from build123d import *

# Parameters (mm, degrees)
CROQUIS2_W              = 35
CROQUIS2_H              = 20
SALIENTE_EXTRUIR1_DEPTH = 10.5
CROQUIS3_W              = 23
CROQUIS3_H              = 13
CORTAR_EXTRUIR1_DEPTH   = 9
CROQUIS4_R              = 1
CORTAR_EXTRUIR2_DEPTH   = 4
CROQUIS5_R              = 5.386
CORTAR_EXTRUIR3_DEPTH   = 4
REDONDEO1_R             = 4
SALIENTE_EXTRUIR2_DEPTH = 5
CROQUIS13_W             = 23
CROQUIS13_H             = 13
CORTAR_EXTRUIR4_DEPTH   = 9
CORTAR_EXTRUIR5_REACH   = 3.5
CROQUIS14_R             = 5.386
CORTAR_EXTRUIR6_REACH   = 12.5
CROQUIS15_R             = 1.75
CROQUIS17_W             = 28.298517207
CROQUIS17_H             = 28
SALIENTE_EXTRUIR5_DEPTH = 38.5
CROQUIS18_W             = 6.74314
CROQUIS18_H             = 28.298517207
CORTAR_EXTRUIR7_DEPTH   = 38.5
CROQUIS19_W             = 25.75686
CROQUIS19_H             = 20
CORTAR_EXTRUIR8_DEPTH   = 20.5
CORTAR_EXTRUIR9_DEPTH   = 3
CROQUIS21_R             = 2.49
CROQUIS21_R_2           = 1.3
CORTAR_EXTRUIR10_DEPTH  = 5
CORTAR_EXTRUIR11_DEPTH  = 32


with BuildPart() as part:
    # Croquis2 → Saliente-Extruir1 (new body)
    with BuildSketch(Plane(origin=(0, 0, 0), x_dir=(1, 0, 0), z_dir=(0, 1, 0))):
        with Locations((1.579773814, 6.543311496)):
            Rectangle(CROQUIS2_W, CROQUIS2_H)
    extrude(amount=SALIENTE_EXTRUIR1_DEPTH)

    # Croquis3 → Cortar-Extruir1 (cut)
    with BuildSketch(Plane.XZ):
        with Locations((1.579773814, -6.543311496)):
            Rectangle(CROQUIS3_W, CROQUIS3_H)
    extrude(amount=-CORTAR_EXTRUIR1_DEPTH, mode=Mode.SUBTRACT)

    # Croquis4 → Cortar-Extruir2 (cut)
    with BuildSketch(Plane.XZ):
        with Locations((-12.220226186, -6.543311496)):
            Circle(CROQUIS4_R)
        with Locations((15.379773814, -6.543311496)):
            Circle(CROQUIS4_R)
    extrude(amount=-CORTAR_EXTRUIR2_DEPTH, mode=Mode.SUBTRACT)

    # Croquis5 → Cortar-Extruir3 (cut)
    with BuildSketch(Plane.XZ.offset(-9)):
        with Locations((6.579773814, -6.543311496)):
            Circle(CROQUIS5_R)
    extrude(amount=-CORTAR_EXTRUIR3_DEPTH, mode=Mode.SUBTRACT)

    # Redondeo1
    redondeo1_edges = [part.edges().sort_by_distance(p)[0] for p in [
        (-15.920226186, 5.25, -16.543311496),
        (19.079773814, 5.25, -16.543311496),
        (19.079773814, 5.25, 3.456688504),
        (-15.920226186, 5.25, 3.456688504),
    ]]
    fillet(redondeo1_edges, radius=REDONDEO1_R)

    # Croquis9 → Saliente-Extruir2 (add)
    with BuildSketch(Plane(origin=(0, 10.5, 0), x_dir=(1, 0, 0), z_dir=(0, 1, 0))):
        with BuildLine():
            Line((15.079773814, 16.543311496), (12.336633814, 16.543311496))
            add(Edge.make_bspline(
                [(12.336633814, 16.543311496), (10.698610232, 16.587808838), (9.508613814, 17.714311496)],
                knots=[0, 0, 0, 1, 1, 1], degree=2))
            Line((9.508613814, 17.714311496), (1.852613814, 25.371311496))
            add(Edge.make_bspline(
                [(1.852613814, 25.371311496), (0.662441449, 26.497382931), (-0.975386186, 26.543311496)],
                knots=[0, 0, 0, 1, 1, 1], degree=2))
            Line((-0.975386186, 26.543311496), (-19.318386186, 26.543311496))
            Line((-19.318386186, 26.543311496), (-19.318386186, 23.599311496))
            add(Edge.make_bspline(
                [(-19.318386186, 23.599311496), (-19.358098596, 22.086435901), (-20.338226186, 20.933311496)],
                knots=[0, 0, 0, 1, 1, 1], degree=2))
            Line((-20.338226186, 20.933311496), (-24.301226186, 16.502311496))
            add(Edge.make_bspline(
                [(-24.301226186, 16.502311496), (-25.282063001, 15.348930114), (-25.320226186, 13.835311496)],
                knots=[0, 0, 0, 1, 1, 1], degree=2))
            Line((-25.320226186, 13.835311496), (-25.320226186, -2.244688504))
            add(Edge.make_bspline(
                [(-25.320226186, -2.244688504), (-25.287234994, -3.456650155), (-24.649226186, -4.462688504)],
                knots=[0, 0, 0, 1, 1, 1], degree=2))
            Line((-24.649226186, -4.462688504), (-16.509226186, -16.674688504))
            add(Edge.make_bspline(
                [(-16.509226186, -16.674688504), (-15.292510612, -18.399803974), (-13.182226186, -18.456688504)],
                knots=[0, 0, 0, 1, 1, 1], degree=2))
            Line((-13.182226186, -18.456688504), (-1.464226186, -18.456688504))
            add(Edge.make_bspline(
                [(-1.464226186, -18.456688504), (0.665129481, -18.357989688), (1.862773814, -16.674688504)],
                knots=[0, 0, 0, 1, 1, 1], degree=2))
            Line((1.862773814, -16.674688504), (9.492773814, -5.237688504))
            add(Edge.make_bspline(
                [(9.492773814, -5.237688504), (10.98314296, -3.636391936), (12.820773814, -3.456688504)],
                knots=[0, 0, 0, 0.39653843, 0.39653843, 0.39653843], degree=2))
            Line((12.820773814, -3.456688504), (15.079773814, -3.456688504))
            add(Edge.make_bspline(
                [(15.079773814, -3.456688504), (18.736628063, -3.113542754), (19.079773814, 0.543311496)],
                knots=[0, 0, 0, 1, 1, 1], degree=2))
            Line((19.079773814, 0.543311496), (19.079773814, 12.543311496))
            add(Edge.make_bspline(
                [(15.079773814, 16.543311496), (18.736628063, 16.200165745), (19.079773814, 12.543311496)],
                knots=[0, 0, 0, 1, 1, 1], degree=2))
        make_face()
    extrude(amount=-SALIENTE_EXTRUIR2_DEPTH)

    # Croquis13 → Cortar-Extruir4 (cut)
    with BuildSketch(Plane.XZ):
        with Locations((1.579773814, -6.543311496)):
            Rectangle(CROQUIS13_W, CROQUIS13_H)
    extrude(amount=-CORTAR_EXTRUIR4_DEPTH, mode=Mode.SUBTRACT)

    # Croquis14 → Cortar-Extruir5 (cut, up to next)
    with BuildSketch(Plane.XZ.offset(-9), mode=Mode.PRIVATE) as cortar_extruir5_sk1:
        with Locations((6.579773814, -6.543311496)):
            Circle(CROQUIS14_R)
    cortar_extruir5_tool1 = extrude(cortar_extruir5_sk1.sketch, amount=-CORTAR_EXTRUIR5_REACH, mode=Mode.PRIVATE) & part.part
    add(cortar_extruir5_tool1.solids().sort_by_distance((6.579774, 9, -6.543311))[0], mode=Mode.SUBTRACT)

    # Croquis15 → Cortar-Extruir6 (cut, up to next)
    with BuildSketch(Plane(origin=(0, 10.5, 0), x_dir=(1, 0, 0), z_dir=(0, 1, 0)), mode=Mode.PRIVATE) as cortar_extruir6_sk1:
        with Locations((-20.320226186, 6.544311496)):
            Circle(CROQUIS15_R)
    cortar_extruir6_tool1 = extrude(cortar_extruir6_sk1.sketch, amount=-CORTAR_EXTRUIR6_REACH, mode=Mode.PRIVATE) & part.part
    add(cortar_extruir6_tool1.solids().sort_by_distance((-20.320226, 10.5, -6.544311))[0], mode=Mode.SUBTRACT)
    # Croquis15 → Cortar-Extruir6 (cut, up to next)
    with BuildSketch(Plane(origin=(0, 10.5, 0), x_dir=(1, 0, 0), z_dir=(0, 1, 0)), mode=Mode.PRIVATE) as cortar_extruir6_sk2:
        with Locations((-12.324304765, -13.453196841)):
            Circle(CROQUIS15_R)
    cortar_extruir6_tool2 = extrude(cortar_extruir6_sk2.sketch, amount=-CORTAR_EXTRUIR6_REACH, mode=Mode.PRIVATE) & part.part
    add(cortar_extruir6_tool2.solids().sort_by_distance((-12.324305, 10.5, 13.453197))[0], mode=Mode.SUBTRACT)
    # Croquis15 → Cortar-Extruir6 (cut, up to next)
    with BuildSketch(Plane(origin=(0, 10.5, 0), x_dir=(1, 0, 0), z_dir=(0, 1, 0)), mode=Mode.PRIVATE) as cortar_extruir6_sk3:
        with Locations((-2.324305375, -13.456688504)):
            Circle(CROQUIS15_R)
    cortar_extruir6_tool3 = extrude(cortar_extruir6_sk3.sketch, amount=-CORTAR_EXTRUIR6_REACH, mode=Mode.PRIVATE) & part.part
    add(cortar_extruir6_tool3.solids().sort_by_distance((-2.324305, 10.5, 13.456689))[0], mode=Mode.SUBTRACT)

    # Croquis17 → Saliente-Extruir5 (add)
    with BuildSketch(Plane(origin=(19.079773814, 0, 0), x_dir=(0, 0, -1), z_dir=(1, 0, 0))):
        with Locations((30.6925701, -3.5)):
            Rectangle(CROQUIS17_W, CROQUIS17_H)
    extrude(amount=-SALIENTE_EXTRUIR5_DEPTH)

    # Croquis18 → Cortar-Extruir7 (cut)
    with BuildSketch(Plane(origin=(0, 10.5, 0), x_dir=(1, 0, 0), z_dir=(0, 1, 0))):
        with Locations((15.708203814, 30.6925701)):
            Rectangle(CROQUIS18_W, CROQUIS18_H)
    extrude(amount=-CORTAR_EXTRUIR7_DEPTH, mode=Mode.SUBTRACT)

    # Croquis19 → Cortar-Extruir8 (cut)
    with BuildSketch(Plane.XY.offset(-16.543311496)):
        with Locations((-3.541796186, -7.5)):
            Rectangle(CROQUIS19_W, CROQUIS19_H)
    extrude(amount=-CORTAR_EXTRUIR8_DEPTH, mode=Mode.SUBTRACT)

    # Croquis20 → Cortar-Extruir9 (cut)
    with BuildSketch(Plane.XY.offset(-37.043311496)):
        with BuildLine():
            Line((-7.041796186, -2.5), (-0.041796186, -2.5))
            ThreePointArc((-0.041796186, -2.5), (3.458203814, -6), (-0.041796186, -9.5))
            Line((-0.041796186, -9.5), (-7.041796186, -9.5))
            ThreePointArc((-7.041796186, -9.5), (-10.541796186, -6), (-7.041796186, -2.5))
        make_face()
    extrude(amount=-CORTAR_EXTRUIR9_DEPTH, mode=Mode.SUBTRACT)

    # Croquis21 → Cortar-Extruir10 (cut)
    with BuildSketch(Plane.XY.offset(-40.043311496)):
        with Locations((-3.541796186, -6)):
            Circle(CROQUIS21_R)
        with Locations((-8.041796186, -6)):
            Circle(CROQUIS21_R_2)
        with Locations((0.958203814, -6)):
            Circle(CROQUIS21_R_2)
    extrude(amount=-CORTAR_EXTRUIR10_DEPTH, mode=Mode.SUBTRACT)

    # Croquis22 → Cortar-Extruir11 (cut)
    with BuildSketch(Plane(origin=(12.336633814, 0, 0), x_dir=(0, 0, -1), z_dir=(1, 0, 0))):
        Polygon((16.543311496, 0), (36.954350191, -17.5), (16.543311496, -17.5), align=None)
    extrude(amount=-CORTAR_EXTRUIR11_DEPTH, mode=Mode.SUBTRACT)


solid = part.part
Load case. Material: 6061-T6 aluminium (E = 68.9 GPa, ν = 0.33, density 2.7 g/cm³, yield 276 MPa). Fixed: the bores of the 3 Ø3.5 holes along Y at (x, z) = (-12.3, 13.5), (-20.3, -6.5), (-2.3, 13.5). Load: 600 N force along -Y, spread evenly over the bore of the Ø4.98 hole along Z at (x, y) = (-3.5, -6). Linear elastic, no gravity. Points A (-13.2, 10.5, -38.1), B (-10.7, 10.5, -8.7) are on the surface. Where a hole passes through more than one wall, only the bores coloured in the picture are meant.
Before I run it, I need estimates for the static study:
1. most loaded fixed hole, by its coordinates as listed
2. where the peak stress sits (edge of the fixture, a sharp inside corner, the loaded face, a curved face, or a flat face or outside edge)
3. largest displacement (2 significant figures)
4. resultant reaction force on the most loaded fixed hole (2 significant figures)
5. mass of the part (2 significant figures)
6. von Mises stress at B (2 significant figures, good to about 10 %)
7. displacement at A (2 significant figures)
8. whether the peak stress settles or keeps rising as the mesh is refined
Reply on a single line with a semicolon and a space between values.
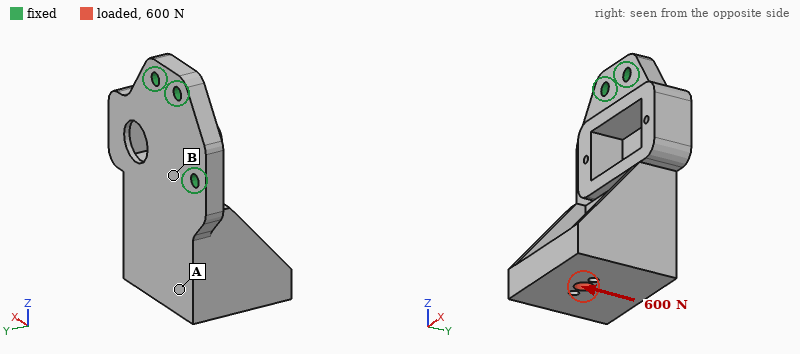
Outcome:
(-20.3, -6.5); edge of the fixture; 0.49 mm; 1.1 kN; 55 g; 71 MPa; 0.25 mm; keeps rising
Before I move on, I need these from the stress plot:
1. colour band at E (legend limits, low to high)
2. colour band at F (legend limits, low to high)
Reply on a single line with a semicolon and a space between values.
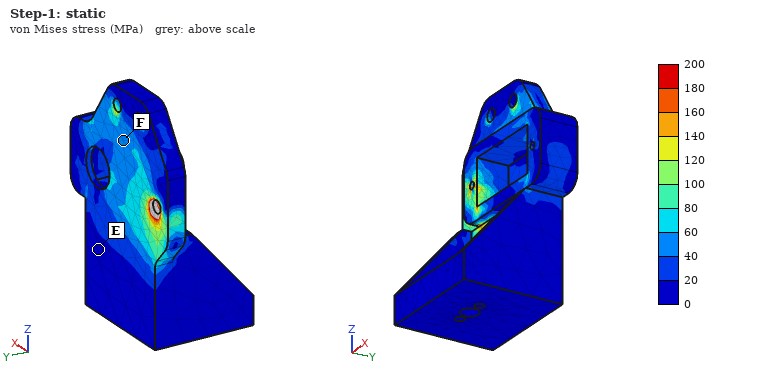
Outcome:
0 to 20 MPa; 40 to 60 MPa
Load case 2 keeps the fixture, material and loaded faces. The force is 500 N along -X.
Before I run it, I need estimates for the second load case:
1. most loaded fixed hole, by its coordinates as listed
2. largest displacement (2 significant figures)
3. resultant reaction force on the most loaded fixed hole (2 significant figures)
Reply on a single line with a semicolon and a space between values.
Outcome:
(-20.3, -6.5); 0.12 mm; 1.0 kN
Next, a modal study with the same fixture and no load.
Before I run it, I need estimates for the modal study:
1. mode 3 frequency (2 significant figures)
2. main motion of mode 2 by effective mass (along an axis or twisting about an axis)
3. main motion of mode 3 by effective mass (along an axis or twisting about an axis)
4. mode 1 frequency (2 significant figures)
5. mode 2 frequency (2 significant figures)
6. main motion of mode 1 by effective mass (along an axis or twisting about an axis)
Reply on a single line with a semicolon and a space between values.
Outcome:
4900 Hz; along X; along X; 1300 Hz; 3100 Hz; along Y
